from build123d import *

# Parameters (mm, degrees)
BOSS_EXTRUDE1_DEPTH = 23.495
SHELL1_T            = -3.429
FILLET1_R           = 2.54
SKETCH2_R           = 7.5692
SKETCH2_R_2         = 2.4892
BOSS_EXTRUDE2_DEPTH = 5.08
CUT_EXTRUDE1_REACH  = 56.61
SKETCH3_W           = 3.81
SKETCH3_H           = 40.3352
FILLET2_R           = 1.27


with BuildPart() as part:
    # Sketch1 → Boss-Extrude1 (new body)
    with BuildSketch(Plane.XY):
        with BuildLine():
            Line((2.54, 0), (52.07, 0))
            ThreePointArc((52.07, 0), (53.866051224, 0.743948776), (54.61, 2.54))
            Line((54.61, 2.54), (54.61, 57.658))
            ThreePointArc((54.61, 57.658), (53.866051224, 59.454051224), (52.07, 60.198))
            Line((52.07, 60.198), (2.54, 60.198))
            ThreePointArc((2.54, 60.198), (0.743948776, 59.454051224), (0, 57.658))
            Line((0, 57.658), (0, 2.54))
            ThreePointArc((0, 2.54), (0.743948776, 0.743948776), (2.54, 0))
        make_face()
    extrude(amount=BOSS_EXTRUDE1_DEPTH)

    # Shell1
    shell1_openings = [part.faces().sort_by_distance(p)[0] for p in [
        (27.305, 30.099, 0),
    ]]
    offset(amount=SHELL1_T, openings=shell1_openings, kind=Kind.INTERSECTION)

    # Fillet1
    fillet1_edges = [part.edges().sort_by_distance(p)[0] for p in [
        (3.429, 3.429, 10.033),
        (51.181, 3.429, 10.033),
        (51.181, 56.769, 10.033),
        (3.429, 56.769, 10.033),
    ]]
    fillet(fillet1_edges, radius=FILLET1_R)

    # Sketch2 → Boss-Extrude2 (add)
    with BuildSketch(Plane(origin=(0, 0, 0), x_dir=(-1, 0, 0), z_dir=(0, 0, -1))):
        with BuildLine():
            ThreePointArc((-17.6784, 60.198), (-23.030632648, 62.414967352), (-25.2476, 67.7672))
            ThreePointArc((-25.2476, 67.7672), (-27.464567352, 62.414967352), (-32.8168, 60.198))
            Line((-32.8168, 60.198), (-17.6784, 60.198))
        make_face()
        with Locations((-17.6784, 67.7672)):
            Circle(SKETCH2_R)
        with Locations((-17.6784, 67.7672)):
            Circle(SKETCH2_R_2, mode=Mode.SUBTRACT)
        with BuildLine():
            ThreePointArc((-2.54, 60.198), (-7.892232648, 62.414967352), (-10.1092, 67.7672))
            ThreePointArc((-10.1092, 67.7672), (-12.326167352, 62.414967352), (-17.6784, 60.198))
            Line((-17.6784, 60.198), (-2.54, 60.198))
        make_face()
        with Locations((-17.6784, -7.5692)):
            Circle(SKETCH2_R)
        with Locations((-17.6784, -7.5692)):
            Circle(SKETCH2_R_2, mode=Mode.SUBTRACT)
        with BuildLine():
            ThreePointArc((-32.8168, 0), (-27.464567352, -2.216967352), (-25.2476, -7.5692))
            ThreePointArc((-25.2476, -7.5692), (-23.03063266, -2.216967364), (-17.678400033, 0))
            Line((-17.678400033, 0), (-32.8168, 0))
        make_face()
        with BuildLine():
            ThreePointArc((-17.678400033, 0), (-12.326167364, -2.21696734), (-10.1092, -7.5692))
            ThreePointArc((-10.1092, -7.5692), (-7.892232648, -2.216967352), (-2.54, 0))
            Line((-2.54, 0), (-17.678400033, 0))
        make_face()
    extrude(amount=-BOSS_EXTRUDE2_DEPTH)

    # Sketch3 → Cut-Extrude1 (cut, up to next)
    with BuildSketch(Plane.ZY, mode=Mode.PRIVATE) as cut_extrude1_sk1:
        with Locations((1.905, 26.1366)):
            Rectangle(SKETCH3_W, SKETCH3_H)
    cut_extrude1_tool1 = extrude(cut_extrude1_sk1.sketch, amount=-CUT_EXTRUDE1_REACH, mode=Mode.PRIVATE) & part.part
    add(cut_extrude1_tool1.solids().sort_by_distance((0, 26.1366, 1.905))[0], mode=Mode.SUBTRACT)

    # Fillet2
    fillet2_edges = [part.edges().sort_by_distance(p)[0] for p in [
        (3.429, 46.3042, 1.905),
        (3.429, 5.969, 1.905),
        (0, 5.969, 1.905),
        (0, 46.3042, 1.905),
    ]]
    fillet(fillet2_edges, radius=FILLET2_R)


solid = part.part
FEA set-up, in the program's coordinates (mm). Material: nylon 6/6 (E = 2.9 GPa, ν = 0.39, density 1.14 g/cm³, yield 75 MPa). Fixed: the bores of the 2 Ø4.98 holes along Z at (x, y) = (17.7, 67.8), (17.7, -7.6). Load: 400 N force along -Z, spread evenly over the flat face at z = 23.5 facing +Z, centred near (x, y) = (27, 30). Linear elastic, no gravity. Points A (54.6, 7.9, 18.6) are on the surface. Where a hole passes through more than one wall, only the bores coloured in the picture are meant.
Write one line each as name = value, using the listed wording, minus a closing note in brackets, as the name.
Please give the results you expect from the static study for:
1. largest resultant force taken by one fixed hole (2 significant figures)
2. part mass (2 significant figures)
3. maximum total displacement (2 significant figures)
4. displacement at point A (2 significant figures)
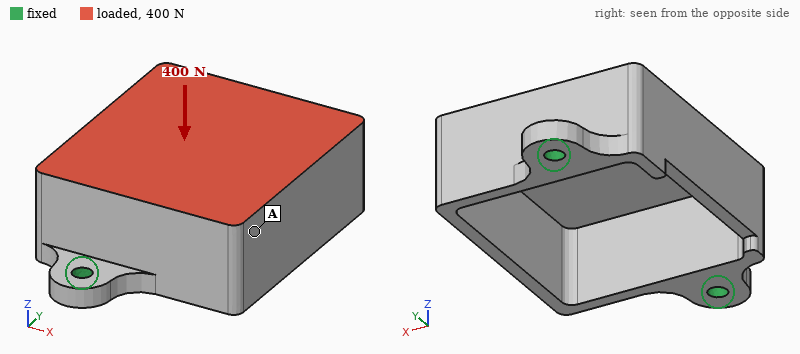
largest resultant force taken by one fixed hole = 210 N
part mass = 32 g
maximum total displacement = 0.90 mm
displacement at point A = 0.85 mm
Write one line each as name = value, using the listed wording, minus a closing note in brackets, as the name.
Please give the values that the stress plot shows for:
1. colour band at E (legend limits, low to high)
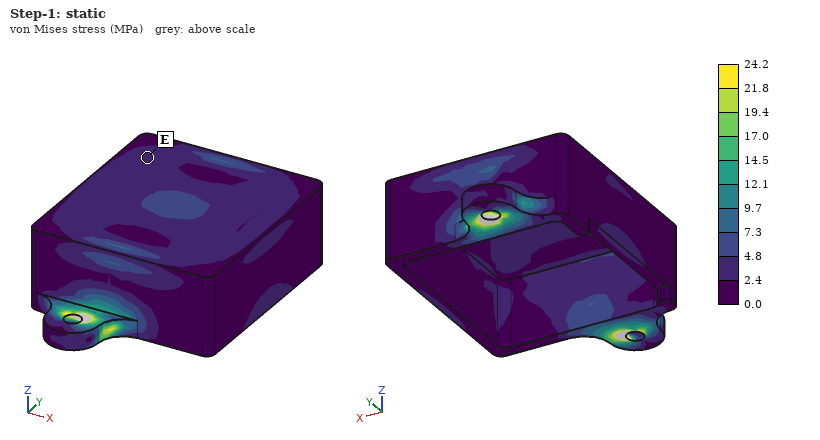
colour band at E = 2.4 to 4.8 MPa
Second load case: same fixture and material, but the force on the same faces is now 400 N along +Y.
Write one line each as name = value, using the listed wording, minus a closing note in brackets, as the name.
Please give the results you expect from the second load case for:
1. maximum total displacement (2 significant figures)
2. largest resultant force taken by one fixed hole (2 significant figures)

maximum total displacement = 0.62 mm
largest resultant force taken by one fixed hole = 240 N
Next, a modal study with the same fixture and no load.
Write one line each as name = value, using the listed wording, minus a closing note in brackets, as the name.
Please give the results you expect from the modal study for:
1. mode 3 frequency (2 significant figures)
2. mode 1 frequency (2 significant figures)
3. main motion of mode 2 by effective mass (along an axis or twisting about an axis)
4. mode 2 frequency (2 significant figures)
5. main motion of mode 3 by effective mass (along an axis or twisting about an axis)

mode 3 frequency = 1800 Hz
mode 1 frequency = 510 Hz
main motion of mode 2 by effective mass = along Y
mode 2 frequency = 810 Hz
main motion of mode 3 by effective mass = along Y
